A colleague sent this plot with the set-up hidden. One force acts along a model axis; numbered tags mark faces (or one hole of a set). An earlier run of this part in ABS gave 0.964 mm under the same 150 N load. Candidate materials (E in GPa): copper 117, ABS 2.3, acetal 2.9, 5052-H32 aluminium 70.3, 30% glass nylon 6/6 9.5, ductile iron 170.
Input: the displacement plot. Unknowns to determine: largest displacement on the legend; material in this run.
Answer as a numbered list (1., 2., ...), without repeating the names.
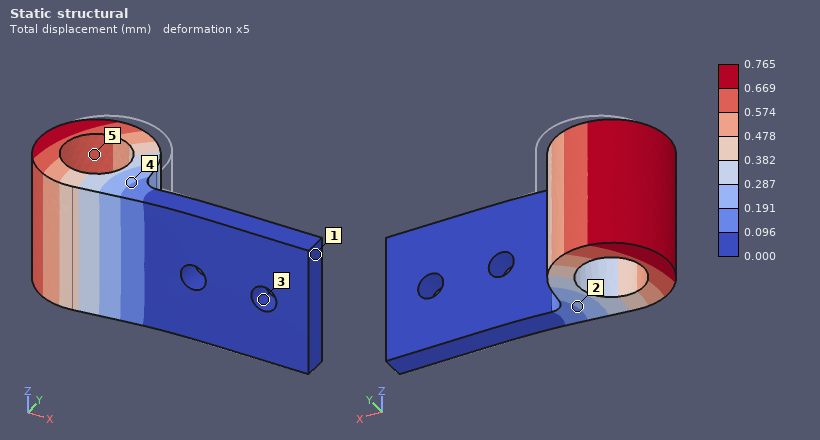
1. 0.765 mm
2. acetal
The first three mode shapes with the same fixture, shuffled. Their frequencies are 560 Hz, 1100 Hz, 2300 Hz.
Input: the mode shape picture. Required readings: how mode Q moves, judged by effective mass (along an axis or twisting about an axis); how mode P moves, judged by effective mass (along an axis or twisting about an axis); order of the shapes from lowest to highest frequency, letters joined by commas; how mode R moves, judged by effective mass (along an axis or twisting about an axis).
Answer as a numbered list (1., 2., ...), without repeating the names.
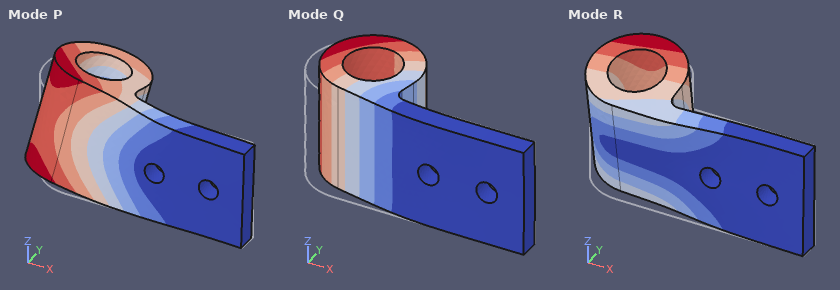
1. along Y
2. along Z
3. Q, R, P
4. along Z
